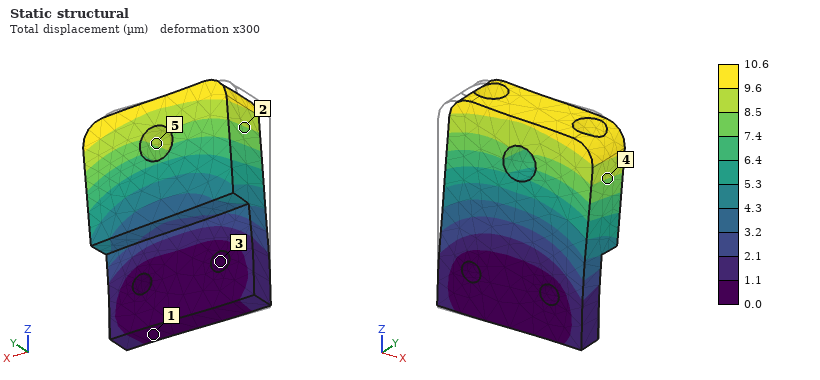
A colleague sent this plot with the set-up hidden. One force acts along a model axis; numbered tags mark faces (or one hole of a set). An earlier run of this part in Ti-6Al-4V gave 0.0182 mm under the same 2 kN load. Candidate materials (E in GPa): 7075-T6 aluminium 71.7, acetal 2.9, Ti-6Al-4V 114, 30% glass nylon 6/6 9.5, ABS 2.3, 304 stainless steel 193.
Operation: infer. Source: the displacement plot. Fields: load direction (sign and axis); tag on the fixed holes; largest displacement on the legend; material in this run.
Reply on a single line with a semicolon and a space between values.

+X; 3; 10.6 µm; 304 stainless steel
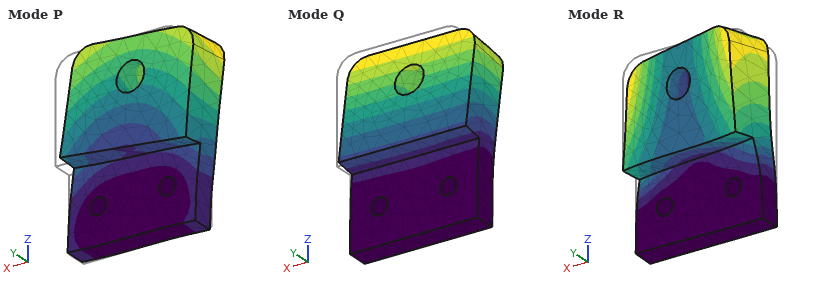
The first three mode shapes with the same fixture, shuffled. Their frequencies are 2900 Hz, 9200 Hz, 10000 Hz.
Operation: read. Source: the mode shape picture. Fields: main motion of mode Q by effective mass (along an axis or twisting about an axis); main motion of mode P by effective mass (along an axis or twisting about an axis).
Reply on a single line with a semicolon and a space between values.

along Y; along X
